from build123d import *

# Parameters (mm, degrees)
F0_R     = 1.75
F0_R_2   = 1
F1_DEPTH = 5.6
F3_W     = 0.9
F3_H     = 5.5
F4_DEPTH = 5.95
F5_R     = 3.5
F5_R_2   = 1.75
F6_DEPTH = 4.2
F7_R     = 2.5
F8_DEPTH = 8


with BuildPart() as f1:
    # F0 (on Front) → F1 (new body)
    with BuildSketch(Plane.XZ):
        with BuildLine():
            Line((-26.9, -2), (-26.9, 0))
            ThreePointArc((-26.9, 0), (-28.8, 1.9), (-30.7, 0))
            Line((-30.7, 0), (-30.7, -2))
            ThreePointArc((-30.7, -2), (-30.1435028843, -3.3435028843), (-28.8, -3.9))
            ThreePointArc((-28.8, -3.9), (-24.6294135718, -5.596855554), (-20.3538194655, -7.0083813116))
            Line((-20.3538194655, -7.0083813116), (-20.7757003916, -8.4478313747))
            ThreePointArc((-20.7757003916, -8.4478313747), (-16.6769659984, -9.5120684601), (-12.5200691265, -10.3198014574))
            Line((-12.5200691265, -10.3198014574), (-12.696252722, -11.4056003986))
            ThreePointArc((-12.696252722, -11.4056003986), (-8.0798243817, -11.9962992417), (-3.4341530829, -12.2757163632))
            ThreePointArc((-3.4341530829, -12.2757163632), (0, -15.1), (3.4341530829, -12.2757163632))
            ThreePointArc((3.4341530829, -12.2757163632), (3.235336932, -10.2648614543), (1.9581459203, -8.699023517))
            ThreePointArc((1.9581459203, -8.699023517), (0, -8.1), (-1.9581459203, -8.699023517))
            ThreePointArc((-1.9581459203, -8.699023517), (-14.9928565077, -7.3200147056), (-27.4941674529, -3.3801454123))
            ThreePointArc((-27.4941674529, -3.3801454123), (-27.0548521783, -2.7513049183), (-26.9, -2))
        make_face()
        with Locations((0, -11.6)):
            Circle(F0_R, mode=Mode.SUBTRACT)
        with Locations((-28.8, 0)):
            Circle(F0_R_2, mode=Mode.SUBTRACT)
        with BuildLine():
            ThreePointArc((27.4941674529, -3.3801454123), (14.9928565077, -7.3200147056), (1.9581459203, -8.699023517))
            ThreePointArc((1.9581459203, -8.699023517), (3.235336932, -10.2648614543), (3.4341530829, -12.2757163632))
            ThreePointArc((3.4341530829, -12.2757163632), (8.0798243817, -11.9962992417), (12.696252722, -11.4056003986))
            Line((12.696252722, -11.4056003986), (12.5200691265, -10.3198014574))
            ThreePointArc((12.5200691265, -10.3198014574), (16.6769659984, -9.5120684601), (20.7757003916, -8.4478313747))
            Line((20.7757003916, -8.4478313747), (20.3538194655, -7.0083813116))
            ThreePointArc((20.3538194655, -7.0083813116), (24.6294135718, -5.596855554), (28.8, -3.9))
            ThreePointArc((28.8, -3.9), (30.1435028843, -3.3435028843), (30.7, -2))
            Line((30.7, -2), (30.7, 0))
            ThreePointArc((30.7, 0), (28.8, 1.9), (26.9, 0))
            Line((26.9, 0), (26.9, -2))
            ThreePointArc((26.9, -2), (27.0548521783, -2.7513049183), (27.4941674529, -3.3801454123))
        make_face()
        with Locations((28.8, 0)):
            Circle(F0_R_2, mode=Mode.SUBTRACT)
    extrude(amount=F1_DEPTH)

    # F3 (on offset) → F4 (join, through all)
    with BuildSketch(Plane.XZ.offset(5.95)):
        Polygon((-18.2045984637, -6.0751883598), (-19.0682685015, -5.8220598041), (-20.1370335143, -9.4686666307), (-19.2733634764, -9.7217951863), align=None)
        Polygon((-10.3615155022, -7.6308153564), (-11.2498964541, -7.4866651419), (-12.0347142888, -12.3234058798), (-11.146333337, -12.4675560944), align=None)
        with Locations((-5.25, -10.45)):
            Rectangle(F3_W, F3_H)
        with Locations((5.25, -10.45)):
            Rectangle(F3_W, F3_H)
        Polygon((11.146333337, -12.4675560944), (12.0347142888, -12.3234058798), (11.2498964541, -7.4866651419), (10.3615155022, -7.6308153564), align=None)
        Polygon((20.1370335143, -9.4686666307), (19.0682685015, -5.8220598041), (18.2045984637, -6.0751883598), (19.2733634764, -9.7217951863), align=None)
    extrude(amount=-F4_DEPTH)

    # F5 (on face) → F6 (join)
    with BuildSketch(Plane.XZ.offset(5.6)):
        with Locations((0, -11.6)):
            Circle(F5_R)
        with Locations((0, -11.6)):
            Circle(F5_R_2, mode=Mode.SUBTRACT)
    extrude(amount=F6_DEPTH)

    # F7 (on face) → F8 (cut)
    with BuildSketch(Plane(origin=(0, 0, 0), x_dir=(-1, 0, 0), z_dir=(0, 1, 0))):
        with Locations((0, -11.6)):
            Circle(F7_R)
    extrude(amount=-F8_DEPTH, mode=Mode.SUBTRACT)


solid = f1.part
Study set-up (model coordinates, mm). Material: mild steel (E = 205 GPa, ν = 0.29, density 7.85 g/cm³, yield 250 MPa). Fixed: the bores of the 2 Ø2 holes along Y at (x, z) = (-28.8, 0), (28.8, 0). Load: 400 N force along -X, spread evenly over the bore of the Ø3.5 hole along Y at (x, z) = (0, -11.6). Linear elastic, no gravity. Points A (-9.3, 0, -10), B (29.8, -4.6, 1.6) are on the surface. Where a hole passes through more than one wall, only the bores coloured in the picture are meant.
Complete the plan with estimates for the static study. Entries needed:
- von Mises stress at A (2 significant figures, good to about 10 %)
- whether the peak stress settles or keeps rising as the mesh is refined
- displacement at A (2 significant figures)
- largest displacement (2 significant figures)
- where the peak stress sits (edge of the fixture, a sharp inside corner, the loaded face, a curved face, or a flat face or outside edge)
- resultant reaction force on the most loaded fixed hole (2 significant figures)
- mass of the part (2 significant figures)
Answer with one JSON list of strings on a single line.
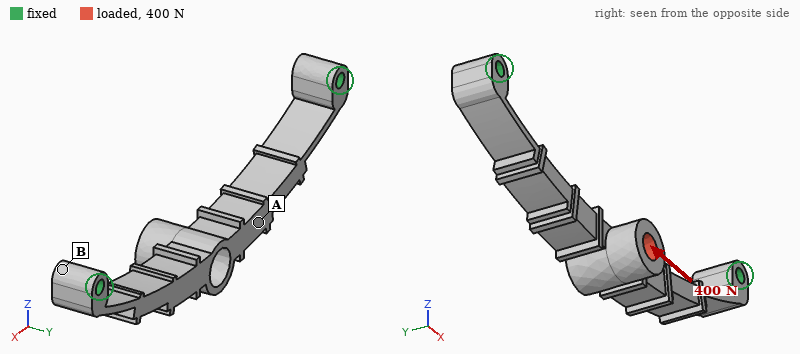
["32 MPa", "keeps rising", "13 µm", "21 µm", "a sharp inside corner", "210 N", "8.9 g"]
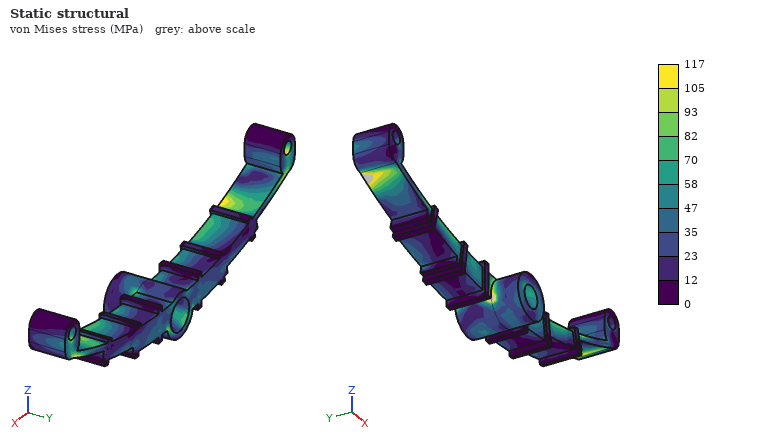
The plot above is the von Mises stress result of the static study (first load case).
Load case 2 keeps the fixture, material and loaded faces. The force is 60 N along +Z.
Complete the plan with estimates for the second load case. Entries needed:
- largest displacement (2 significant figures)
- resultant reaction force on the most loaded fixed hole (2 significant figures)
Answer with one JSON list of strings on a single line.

["62 µm", "88 N"]
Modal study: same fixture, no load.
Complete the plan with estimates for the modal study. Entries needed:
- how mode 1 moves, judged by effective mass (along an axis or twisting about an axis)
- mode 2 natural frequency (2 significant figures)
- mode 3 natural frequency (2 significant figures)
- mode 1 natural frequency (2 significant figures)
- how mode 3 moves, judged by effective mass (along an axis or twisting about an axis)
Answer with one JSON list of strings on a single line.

["along Y", "5800 Hz", "6300 Hz", "3100 Hz", "along Z"]
